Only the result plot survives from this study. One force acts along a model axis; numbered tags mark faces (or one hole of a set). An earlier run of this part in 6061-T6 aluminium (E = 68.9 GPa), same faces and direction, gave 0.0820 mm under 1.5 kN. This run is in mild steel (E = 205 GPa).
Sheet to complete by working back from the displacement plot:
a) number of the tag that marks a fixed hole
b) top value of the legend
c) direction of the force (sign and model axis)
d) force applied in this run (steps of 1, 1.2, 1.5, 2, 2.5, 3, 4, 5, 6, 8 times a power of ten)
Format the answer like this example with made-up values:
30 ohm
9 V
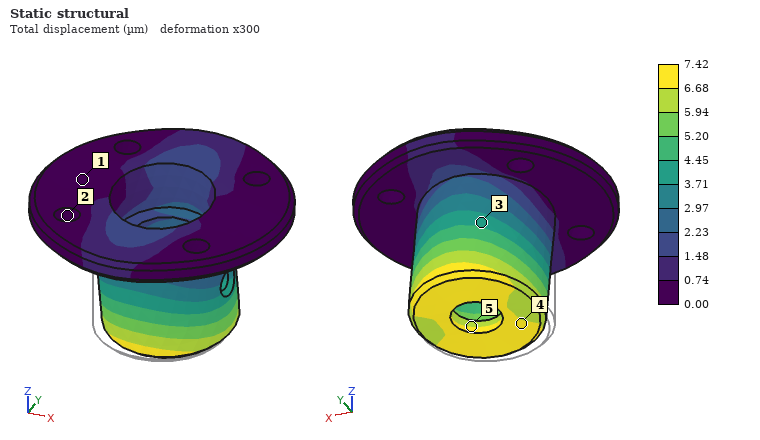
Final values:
2
7.42 µm
+Y
400 N
